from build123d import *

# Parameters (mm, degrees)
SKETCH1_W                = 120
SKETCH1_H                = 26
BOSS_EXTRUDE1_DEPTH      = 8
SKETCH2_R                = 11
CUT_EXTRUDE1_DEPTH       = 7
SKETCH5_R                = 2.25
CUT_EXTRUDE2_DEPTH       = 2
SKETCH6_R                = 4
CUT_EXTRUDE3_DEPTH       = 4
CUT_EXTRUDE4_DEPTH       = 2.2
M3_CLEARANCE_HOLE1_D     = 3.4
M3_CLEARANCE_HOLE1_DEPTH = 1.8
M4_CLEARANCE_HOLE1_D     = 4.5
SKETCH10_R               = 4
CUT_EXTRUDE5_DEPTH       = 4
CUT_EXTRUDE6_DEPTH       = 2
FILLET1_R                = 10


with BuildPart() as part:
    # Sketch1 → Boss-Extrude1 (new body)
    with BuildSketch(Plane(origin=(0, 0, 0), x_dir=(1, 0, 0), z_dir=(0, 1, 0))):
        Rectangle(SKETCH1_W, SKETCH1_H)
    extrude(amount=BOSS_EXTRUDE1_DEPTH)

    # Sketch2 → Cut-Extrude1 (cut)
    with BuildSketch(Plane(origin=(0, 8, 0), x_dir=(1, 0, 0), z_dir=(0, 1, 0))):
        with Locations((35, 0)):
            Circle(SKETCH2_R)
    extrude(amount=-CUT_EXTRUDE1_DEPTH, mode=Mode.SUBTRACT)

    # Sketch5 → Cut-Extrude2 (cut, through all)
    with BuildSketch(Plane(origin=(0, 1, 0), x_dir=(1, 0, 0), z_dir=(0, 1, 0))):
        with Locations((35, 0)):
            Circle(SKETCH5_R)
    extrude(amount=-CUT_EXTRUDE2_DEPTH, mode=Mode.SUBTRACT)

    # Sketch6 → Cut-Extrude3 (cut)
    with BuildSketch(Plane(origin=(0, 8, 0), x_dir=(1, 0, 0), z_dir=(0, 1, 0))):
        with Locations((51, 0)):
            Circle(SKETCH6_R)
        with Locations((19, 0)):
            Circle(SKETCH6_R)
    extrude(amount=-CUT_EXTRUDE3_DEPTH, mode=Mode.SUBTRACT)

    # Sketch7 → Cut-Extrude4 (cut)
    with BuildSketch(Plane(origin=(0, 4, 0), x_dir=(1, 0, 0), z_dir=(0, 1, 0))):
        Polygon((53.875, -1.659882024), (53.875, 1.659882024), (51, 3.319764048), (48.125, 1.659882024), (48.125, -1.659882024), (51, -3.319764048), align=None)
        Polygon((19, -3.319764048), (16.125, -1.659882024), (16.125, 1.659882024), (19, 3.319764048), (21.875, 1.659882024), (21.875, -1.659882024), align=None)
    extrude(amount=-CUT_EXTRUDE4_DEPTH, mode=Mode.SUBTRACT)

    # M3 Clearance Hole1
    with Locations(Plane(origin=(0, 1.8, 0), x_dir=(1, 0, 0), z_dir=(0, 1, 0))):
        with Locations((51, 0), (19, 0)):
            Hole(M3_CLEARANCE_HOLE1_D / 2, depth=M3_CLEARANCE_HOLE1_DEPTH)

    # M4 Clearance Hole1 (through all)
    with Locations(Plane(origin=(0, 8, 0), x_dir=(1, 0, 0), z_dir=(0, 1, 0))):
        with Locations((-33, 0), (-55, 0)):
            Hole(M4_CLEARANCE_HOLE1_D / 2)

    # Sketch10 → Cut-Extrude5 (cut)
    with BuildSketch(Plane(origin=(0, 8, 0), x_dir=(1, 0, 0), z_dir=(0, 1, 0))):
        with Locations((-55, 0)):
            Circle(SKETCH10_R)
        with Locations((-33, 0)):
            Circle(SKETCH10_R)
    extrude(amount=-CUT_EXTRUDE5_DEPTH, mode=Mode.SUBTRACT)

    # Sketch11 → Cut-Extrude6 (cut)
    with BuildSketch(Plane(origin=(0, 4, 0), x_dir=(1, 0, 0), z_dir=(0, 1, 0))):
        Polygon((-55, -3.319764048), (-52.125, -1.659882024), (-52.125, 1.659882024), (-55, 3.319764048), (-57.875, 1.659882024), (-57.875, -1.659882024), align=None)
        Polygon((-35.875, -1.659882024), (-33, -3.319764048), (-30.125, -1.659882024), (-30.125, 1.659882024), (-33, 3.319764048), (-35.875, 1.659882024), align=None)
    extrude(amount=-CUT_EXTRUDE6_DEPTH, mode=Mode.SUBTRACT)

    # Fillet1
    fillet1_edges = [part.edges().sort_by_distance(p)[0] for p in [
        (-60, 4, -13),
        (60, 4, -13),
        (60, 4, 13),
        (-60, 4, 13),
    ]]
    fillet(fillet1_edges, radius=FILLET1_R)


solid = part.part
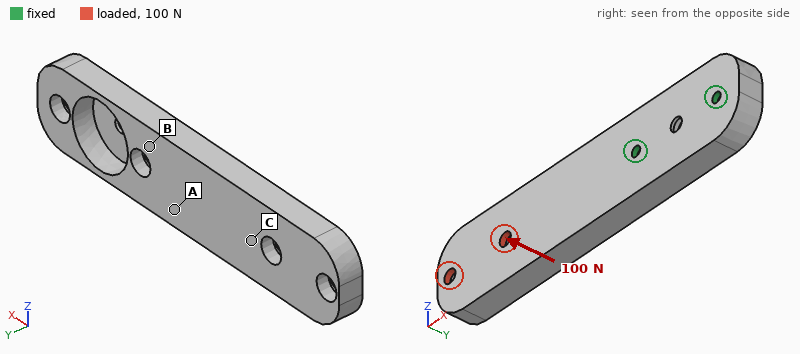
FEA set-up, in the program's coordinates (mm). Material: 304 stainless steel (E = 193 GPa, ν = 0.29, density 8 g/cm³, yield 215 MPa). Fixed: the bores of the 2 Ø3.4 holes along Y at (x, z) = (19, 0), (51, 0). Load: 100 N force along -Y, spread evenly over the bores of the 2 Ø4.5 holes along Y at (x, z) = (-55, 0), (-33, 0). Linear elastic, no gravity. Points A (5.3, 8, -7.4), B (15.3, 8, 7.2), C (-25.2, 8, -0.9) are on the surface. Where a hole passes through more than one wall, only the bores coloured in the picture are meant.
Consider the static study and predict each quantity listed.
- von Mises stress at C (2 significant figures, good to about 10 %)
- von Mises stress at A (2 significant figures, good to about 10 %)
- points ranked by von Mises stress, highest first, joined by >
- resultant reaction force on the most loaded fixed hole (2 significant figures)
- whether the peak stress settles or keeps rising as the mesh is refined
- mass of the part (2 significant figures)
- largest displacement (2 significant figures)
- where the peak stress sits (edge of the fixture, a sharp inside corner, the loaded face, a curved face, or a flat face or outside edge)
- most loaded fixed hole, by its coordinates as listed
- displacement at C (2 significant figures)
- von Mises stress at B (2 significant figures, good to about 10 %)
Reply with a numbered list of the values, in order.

1. 5.1 MPa
2. 18 MPa
3. B > A > C
4. 390 N
5. keeps rising
6. 160 g
7. 98 µm
8. edge of the fixture
9. (19, 0)
10. 47 µm
11. 25 MPa
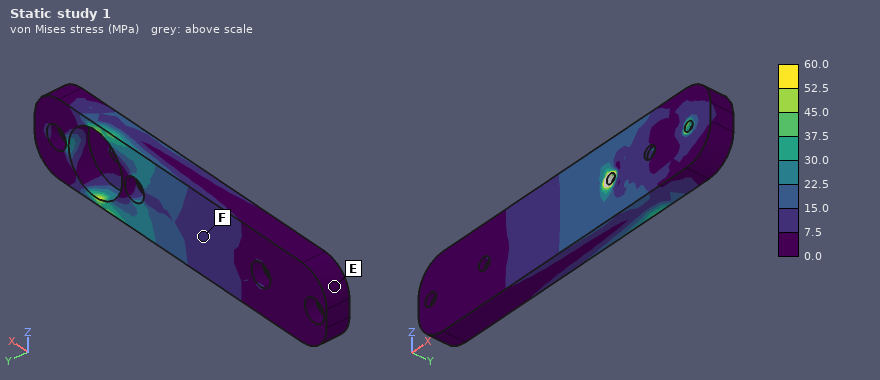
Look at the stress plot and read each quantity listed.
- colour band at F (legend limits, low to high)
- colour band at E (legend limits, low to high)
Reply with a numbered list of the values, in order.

1. 7.5 to 15.0 MPa
2. 0.0 to 7.5 MPa
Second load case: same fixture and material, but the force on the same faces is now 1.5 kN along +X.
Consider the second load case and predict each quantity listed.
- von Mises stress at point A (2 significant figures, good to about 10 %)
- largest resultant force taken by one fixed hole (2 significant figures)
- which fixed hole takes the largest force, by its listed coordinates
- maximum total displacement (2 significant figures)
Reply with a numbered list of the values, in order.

1. 9.1 MPa
2. 1.2 kN
3. (19, 0)
4. 64 µm
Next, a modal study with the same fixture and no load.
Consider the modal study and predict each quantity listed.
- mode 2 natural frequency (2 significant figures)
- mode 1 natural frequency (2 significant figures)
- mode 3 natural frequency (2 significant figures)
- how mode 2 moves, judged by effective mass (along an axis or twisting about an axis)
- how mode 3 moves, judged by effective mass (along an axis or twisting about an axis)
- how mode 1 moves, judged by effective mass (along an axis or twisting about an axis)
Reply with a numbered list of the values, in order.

1. 1800 Hz
2. 780 Hz
3. 2700 Hz
4. along Z
5. twisting about X
6. along Y
